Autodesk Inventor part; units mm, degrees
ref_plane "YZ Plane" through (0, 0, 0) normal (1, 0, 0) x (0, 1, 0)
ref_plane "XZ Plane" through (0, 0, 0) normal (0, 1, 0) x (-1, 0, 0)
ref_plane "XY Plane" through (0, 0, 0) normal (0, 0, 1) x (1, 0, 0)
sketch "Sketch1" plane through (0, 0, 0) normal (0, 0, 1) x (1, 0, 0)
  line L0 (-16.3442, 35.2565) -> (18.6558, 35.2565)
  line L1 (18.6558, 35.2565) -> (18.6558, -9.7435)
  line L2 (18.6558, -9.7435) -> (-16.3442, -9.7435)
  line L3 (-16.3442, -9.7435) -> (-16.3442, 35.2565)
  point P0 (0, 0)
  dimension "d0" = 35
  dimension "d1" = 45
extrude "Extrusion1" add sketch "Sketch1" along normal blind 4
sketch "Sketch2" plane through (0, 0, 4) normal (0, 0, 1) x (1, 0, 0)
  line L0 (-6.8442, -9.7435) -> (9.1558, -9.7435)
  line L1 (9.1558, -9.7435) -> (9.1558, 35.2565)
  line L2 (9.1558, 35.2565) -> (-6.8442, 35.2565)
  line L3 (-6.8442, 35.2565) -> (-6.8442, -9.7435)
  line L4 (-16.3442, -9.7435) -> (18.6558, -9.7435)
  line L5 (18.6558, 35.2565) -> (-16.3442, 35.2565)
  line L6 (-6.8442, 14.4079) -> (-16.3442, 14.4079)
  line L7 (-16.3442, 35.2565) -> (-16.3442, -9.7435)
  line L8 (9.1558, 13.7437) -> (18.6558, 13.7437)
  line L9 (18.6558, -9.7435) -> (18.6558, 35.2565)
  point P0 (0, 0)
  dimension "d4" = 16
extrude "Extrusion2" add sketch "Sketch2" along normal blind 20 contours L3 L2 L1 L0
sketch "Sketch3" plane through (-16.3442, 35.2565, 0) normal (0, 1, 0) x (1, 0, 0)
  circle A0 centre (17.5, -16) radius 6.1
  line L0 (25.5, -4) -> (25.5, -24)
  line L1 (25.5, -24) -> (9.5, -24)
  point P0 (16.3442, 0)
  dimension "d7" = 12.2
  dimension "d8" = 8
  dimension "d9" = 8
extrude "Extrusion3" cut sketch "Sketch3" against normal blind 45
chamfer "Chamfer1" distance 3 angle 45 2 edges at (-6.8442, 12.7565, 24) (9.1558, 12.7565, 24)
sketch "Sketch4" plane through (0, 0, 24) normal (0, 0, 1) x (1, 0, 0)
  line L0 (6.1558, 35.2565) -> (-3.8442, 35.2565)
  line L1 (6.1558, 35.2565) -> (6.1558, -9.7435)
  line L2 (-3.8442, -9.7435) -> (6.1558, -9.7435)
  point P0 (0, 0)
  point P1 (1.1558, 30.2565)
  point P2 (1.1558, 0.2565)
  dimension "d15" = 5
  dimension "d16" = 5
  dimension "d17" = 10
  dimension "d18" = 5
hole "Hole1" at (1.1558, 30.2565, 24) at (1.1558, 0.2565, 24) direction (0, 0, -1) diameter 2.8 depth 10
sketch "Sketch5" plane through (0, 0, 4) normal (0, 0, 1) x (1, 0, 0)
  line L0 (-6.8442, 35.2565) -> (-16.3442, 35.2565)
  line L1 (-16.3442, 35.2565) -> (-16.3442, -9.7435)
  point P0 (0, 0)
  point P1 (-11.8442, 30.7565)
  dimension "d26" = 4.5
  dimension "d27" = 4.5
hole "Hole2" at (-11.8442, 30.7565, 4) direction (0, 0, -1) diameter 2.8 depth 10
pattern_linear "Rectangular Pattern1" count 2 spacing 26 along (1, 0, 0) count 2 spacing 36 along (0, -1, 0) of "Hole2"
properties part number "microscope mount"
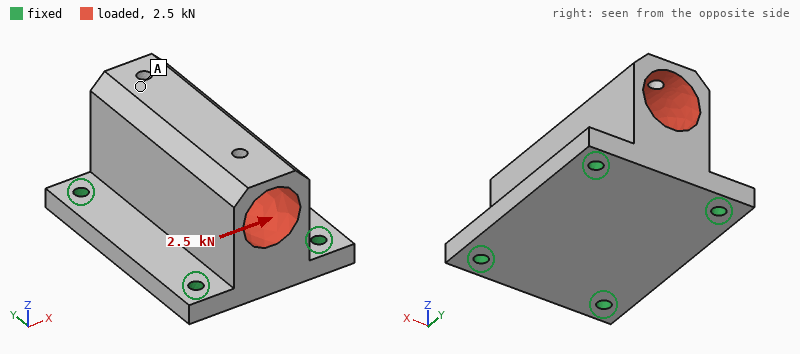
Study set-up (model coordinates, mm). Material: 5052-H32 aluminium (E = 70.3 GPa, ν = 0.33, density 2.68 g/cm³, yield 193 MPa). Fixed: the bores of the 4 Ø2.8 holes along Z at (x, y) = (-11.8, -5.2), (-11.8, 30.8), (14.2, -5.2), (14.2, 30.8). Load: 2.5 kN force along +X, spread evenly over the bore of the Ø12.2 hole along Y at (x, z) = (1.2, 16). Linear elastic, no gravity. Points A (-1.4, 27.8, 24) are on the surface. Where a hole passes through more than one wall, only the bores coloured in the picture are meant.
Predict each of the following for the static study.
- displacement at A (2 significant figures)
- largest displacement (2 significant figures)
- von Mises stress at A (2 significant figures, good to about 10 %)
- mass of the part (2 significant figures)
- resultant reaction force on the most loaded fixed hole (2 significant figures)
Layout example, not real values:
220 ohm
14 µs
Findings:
44 µm
45 µm
20 MPa
40 g
1.0 kN
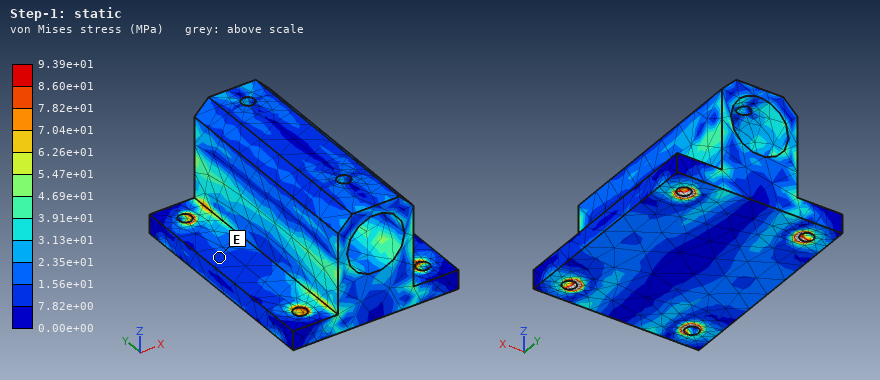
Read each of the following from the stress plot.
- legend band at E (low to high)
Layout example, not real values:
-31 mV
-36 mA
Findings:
7.82e+00 to 1.56e+01 MPa
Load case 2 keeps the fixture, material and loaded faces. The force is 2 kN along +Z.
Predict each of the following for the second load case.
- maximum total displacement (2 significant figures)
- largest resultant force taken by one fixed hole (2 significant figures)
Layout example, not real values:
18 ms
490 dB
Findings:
10 µm
530 N
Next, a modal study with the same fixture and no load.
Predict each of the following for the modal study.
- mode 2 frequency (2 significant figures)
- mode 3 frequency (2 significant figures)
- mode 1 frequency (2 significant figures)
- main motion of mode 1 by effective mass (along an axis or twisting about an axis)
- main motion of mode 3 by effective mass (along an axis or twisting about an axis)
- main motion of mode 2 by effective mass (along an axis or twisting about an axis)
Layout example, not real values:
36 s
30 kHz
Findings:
14 kHz
15 kHz
11 kHz
along X
along Y
along Z
